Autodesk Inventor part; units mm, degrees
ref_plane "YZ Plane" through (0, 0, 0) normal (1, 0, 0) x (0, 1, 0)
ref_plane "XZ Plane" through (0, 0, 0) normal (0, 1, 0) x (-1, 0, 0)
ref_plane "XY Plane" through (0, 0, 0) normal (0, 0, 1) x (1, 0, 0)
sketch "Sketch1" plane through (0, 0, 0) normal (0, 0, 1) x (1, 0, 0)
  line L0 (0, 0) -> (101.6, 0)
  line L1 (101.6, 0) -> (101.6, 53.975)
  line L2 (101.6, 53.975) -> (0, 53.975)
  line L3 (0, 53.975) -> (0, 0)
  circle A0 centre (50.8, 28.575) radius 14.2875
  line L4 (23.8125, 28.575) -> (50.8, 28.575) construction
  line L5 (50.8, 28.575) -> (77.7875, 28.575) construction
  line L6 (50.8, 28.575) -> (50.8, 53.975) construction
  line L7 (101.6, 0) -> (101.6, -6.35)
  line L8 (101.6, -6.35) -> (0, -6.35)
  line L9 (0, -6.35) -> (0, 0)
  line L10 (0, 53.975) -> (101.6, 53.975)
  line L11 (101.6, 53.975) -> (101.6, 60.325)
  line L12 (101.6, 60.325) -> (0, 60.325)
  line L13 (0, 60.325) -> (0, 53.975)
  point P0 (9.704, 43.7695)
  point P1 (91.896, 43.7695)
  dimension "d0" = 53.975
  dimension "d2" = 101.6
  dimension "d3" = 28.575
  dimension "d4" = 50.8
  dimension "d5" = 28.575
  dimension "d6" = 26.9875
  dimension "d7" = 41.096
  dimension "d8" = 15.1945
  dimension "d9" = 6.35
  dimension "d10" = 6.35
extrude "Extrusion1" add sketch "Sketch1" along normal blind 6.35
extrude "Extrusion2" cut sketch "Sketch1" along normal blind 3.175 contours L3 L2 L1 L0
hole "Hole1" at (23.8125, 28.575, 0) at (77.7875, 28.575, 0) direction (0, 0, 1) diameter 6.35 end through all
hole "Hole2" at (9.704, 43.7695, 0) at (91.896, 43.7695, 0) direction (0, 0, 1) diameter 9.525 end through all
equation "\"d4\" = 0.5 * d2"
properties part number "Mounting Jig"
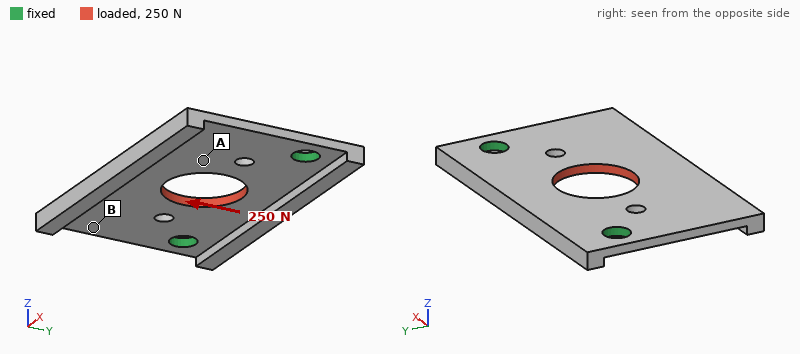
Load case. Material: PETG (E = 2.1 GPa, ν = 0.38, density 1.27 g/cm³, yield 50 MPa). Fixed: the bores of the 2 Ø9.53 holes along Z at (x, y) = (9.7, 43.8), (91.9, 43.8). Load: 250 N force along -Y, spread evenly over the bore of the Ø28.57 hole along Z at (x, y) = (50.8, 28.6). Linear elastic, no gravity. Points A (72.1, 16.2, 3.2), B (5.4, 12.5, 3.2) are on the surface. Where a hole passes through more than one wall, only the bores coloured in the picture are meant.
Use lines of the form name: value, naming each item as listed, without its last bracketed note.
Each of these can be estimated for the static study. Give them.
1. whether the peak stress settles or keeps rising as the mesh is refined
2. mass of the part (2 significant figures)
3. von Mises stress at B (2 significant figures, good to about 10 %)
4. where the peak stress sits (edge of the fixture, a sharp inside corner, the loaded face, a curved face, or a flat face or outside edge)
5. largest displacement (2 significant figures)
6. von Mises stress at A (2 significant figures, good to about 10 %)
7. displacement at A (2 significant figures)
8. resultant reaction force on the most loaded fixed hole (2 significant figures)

whether the peak stress settles or keeps rising as the mesh is refined: keeps rising
mass of the part: 29 g
von Mises stress at B: 0.60 MPa
where the peak stress sits: edge of the fixture
largest displacement: 82 µm
von Mises stress at A: 1.4 MPa
displacement at A: 39 µm
resultant reaction force on the most loaded fixed hole: 130 N
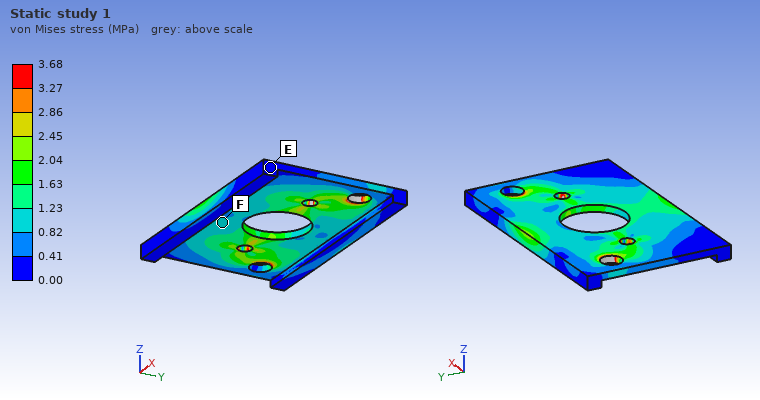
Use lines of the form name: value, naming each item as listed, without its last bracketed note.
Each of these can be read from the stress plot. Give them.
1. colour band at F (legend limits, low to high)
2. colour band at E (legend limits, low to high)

colour band at F: 0.82 to 1.23 MPa
colour band at E: 0.00 to 0.41 MPa
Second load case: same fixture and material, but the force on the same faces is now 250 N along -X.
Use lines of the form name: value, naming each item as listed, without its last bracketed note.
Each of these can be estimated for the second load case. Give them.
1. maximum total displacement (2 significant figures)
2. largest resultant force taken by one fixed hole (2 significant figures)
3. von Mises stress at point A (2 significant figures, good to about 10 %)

maximum total displacement: 52 µm
largest resultant force taken by one fixed hole: 130 N
von Mises stress at point A: 1.2 MPa
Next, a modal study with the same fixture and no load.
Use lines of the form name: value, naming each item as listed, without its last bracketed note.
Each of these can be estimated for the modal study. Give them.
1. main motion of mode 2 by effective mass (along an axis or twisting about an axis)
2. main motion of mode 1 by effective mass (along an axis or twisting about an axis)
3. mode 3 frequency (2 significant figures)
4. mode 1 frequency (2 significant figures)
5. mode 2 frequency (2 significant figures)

main motion of mode 2 by effective mass: twisting about Y
main motion of mode 1 by effective mass: along Z
mode 3 frequency: 820 Hz
mode 1 frequency: 200 Hz
mode 2 frequency: 400 Hz
